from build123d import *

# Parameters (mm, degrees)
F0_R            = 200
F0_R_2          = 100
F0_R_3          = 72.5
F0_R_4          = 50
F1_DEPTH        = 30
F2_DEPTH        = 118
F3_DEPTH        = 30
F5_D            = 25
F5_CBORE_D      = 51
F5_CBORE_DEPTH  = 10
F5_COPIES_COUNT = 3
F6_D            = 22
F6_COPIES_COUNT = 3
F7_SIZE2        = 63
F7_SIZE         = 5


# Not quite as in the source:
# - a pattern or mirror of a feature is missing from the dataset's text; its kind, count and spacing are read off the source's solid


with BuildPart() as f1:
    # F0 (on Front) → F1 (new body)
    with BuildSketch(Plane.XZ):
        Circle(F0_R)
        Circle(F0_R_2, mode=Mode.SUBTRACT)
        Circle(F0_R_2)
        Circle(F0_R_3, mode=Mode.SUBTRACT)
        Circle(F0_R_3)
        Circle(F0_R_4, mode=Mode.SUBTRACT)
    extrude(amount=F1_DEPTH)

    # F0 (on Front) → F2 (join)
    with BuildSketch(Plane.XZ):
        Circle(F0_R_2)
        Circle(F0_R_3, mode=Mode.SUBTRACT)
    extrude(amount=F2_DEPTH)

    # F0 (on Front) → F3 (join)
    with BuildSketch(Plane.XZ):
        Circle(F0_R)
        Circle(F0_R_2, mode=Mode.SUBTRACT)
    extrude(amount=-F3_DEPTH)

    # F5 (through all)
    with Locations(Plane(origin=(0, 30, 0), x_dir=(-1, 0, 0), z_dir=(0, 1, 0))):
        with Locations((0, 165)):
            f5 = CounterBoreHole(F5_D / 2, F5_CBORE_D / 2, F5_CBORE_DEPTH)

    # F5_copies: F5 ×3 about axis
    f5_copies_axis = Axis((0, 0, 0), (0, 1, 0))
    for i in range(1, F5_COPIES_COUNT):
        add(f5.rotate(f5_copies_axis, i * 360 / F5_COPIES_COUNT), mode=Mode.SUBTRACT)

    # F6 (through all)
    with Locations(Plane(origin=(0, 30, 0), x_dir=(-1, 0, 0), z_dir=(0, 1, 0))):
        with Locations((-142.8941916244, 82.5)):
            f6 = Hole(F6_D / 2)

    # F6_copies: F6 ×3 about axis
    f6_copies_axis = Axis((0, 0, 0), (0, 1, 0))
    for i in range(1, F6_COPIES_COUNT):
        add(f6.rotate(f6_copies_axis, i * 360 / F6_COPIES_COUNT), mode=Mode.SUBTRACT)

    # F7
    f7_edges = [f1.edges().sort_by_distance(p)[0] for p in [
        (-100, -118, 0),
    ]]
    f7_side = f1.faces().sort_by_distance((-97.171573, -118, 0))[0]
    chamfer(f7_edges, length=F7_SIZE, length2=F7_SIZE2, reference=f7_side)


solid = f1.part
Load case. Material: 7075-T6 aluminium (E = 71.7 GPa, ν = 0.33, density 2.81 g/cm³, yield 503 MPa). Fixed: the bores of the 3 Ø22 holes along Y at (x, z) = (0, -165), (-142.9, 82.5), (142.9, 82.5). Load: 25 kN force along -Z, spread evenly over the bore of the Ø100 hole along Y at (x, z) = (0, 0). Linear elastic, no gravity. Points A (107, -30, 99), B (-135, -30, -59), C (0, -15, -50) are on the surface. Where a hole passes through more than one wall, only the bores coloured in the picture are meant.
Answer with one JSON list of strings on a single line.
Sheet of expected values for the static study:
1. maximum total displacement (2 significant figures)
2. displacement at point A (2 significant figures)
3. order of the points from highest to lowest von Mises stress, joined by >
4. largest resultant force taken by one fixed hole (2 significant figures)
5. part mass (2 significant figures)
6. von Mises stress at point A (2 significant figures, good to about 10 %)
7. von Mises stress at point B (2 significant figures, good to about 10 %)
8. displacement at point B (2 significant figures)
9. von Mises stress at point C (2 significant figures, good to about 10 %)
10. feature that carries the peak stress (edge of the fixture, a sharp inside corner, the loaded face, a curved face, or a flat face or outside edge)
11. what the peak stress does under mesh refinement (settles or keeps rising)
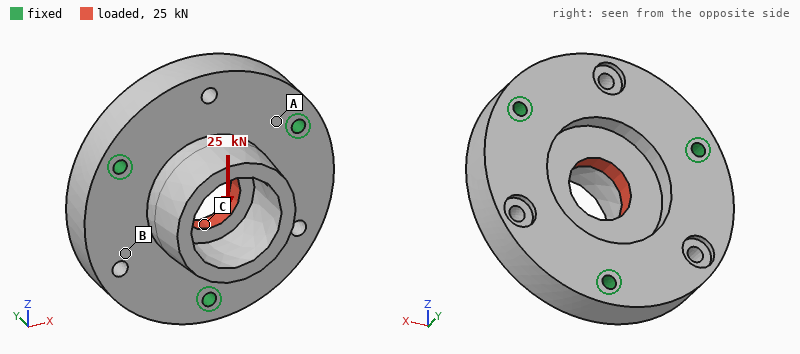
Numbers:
["6.4 µm", "2.0 µm", "C > A > B", "8.5 kN", "21 kg", "1.7 MPa", "0.79 MPa", "2.4 µm", "3.2 MPa", "edge of the fixture", "keeps rising"]
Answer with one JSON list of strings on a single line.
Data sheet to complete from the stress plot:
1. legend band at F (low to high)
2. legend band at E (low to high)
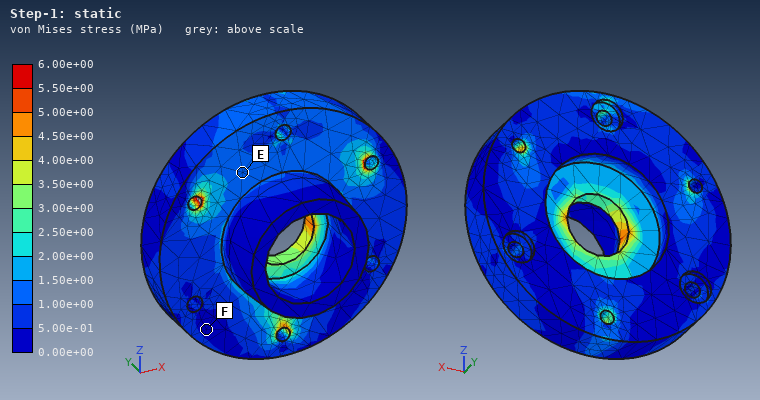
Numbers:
["0.00e+00 to 5.00e-01 MPa", "1.00e+00 to 1.50e+00 MPa"]
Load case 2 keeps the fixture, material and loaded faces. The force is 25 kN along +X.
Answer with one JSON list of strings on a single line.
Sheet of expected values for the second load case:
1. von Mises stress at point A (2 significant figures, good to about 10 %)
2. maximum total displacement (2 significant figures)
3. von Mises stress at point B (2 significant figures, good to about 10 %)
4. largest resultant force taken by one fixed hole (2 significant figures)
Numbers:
["1.4 MPa", "6.1 µm", "1.3 MPa", "8.5 kN"]
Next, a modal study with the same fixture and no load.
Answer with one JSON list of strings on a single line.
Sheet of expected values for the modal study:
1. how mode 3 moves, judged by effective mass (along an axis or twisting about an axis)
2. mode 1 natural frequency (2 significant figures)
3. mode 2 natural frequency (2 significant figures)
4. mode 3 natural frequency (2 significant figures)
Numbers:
["along Y", "1900 Hz", "1900 Hz", "2200 Hz"]
